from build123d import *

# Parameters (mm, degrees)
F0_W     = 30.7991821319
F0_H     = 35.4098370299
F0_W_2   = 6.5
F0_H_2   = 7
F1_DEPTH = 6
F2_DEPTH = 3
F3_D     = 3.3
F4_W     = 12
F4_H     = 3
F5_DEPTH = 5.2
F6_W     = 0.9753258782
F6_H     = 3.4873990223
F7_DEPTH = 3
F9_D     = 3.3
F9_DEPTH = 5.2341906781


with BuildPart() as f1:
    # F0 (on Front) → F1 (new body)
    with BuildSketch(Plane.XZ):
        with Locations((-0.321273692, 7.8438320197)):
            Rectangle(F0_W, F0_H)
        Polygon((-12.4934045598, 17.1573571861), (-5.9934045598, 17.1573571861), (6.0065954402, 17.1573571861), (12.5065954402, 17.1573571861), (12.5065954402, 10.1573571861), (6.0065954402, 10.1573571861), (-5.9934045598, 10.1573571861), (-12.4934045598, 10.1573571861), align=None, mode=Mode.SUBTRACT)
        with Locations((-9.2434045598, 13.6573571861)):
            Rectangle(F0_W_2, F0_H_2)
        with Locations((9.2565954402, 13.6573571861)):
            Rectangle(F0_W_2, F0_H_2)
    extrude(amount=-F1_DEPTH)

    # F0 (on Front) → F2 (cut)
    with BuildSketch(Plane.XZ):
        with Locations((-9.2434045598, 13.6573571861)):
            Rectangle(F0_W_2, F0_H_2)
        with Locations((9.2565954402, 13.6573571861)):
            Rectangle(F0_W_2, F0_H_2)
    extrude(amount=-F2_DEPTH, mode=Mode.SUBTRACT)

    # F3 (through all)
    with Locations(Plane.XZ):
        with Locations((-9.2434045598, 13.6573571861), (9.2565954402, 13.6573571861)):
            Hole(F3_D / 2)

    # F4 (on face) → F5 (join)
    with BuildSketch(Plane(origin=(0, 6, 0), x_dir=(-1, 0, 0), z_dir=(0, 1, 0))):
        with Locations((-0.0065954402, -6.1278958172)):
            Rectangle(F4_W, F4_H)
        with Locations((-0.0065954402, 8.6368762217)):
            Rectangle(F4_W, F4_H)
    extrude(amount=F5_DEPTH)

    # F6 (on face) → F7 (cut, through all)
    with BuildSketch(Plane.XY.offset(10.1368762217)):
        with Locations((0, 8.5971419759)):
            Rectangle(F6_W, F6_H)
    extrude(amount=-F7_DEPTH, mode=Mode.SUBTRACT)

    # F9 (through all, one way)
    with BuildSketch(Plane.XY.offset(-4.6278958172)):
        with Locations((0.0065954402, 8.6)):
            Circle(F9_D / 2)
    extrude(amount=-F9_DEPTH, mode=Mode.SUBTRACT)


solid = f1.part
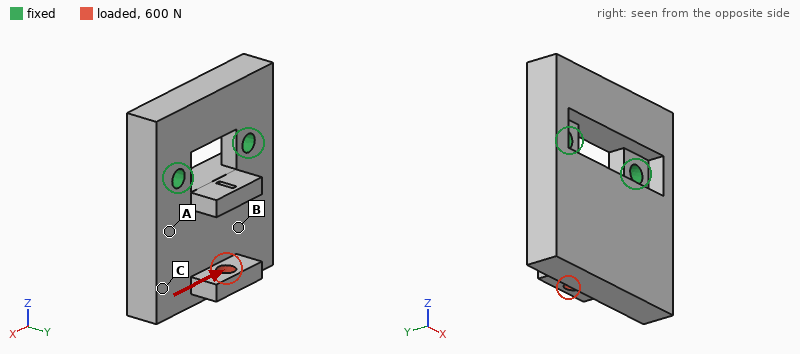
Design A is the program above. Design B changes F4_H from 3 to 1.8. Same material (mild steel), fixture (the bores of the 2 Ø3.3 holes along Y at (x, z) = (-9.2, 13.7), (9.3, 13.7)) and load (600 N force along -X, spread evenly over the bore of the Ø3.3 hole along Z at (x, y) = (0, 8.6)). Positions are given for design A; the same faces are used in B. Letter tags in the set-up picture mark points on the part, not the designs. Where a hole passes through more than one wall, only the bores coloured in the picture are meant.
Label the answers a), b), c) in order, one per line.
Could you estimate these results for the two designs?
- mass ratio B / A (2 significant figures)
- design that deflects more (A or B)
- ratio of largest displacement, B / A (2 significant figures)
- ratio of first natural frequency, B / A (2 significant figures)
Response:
a) 0.98
b) B
c) 1.1
d) 1.0
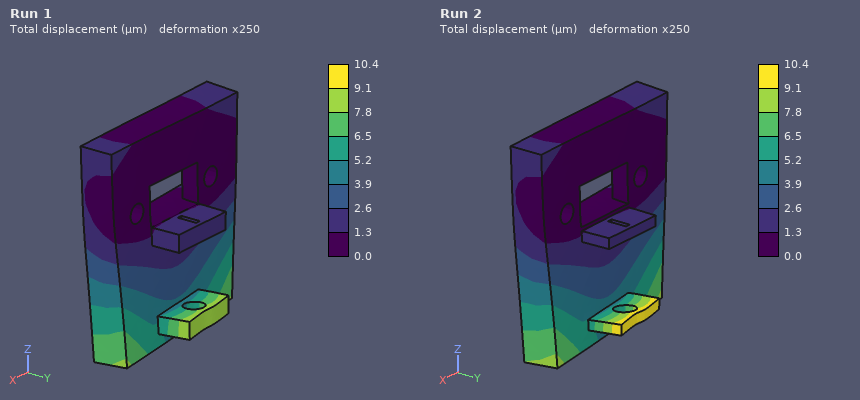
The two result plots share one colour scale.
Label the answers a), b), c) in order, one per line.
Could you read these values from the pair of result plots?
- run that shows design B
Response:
a) Run 2
